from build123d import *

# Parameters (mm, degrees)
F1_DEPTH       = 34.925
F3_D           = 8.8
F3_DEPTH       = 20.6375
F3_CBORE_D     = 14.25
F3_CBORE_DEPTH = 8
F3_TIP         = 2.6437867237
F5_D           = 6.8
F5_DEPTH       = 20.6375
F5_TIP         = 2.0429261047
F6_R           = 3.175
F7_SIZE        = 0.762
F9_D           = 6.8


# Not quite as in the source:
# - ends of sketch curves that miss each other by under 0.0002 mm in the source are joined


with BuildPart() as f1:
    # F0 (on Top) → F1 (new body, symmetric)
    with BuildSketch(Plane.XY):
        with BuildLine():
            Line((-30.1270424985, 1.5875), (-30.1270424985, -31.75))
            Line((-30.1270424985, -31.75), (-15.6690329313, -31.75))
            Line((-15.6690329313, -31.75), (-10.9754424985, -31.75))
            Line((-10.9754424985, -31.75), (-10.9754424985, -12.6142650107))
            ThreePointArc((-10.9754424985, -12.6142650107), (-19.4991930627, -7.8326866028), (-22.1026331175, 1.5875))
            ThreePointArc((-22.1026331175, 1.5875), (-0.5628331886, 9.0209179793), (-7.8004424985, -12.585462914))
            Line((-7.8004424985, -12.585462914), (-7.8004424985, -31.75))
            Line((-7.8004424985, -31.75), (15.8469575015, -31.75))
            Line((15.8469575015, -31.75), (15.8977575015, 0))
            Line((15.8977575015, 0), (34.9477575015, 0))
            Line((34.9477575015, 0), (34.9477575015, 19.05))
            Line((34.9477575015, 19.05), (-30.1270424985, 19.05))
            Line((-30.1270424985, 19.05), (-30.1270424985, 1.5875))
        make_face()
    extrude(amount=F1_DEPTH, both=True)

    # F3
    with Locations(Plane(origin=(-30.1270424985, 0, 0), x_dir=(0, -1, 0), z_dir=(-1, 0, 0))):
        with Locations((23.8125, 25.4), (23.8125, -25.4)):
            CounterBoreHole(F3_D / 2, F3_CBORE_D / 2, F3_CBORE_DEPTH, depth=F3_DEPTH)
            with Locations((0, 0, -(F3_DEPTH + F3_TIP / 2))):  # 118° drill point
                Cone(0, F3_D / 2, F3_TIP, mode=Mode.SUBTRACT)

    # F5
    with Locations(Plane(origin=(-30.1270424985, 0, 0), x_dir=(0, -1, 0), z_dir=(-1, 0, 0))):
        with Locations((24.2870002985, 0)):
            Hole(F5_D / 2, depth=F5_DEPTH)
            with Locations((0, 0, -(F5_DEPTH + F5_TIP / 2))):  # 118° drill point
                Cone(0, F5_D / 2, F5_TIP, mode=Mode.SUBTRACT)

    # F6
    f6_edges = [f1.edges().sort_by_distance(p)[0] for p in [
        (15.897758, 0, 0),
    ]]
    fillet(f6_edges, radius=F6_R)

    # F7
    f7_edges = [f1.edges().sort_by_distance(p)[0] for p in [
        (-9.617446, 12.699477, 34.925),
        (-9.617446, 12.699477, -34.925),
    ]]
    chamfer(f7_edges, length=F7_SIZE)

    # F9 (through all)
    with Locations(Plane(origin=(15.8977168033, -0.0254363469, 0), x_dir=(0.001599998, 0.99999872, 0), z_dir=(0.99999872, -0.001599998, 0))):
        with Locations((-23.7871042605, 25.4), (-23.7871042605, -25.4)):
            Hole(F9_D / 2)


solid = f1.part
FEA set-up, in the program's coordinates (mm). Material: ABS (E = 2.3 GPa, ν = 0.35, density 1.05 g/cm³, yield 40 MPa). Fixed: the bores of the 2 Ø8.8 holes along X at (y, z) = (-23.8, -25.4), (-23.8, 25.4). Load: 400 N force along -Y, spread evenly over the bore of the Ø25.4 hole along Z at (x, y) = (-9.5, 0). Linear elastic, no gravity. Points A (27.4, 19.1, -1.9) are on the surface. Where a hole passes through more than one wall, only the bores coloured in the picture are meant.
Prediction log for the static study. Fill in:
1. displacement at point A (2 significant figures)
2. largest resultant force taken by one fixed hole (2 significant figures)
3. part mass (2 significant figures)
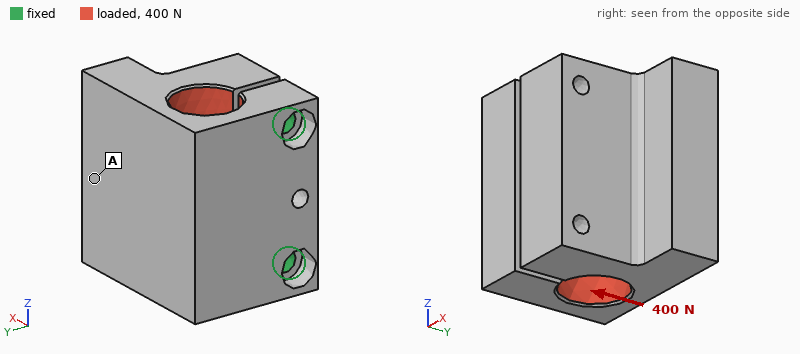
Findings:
1.1 mm
210 N
150 g
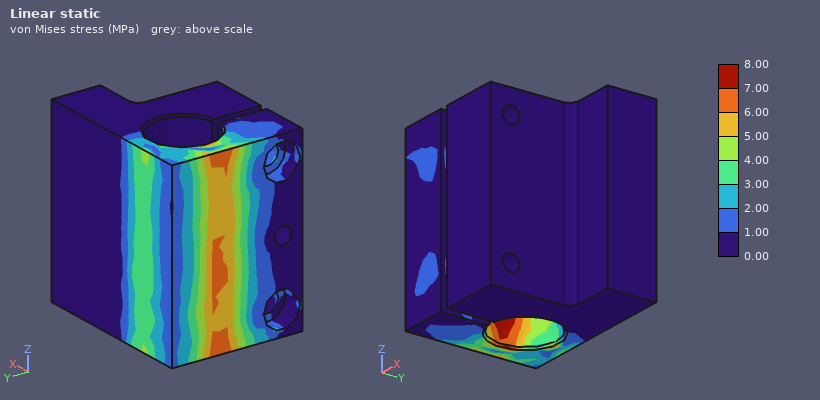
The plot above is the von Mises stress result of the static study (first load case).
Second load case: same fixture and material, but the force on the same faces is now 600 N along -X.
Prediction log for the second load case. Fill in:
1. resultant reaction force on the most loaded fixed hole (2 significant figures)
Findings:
310 N
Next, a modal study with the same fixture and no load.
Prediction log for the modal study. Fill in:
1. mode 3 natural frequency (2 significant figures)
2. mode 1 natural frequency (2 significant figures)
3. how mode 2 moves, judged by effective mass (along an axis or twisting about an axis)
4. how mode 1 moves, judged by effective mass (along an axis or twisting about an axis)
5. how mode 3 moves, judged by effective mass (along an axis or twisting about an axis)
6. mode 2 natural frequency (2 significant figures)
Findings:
440 Hz
180 Hz
along Z
along Y
along X
320 Hz
